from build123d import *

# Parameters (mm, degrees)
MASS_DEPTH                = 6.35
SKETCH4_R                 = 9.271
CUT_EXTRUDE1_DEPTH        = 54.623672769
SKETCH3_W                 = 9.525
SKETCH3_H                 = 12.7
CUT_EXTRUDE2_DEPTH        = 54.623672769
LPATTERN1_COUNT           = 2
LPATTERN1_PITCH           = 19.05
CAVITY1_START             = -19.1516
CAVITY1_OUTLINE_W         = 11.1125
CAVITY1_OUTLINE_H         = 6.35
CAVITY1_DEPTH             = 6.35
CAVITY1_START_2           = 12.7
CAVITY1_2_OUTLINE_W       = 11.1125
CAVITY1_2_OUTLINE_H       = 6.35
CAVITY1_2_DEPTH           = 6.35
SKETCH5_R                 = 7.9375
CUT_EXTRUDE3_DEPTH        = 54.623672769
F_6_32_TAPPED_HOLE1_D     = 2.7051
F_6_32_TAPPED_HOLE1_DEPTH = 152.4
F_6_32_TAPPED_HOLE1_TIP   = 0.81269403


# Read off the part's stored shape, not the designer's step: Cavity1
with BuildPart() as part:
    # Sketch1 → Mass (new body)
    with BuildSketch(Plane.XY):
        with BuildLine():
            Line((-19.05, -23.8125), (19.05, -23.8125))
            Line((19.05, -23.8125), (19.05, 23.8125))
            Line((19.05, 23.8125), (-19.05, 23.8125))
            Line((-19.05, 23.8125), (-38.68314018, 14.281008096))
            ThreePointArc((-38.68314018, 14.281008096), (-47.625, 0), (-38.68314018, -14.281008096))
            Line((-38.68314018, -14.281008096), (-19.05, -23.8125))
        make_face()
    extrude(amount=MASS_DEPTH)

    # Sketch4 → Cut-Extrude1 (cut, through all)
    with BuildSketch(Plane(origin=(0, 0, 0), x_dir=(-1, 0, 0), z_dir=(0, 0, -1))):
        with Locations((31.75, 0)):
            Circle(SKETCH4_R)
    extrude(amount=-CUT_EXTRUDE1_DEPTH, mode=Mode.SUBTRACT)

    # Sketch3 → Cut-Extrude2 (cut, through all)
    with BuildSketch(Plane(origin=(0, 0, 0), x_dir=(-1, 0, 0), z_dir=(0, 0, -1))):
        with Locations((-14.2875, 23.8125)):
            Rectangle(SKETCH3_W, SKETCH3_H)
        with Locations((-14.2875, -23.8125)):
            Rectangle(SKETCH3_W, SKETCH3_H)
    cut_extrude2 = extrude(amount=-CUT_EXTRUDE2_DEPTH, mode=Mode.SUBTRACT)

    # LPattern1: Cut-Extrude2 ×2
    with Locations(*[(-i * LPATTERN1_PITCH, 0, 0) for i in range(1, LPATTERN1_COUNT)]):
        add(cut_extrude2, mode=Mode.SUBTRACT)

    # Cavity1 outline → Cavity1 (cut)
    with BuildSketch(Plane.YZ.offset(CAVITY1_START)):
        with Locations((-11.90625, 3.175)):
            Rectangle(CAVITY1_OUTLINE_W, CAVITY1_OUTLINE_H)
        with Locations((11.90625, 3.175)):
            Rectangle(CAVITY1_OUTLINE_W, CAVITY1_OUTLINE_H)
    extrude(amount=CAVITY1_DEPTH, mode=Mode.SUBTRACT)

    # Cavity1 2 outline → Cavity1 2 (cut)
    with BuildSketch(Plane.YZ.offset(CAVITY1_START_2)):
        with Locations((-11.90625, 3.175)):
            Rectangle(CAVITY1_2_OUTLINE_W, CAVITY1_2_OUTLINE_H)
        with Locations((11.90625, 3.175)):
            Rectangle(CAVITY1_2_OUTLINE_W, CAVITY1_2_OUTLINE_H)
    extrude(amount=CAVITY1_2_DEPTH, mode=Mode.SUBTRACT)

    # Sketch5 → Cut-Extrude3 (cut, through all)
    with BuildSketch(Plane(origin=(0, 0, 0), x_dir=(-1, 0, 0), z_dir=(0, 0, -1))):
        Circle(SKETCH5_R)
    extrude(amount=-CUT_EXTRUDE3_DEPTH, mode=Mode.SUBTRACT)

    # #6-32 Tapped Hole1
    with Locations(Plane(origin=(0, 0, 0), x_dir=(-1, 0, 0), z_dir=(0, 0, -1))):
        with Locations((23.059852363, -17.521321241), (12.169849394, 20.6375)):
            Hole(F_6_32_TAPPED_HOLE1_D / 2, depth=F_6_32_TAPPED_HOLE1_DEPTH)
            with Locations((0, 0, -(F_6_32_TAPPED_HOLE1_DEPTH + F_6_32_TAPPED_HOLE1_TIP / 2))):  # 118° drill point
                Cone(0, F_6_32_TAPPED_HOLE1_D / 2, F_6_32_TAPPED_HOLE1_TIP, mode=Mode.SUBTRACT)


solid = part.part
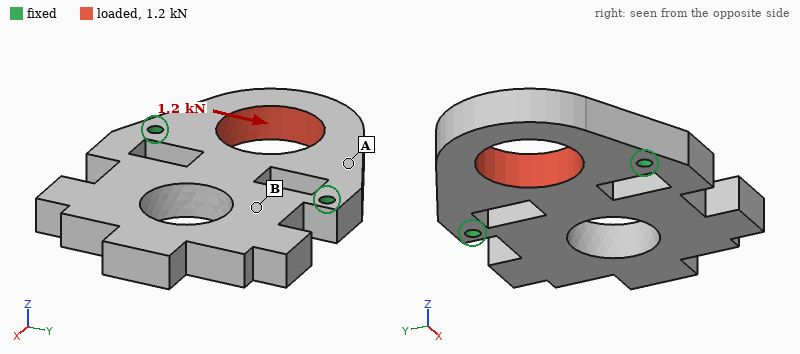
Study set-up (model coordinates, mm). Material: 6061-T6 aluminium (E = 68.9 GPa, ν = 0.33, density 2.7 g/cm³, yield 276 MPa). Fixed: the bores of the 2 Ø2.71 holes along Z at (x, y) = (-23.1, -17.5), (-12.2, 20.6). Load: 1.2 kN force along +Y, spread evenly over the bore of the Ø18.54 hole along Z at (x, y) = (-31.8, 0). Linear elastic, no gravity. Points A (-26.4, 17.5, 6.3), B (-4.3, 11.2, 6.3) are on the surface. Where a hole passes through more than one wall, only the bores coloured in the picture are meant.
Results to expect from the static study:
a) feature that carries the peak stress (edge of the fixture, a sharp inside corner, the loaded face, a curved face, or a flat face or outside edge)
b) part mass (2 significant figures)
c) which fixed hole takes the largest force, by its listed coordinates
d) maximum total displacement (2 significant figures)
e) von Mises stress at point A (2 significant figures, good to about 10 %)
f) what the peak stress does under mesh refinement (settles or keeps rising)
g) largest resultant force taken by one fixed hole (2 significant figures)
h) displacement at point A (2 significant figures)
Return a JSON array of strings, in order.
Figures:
["edge of the fixture", "30 g", "(-23.1, -17.5)", "13 µm", "9.1 MPa", "keeps rising", "880 N", "5.6 µm"]
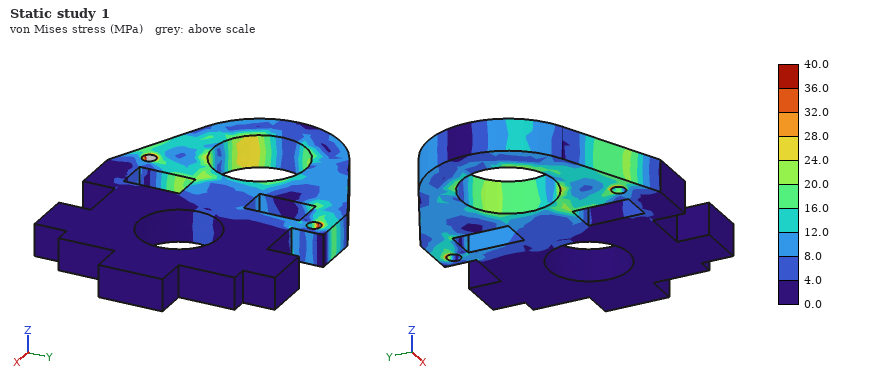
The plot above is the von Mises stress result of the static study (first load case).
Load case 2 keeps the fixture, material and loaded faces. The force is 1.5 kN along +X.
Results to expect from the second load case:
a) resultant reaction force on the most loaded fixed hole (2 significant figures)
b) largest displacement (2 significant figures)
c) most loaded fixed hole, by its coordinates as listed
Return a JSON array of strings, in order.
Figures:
["810 N", "6.1 µm", "(-23.1, -17.5)"]
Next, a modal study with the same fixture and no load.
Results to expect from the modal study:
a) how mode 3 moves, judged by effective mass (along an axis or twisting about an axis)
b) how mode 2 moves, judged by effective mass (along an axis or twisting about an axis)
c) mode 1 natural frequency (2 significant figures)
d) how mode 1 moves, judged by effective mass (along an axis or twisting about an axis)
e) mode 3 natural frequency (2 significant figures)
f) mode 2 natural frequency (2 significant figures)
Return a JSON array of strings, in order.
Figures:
["twisting about X", "along Z", "2600 Hz", "along Z", "6700 Hz", "5500 Hz"]
